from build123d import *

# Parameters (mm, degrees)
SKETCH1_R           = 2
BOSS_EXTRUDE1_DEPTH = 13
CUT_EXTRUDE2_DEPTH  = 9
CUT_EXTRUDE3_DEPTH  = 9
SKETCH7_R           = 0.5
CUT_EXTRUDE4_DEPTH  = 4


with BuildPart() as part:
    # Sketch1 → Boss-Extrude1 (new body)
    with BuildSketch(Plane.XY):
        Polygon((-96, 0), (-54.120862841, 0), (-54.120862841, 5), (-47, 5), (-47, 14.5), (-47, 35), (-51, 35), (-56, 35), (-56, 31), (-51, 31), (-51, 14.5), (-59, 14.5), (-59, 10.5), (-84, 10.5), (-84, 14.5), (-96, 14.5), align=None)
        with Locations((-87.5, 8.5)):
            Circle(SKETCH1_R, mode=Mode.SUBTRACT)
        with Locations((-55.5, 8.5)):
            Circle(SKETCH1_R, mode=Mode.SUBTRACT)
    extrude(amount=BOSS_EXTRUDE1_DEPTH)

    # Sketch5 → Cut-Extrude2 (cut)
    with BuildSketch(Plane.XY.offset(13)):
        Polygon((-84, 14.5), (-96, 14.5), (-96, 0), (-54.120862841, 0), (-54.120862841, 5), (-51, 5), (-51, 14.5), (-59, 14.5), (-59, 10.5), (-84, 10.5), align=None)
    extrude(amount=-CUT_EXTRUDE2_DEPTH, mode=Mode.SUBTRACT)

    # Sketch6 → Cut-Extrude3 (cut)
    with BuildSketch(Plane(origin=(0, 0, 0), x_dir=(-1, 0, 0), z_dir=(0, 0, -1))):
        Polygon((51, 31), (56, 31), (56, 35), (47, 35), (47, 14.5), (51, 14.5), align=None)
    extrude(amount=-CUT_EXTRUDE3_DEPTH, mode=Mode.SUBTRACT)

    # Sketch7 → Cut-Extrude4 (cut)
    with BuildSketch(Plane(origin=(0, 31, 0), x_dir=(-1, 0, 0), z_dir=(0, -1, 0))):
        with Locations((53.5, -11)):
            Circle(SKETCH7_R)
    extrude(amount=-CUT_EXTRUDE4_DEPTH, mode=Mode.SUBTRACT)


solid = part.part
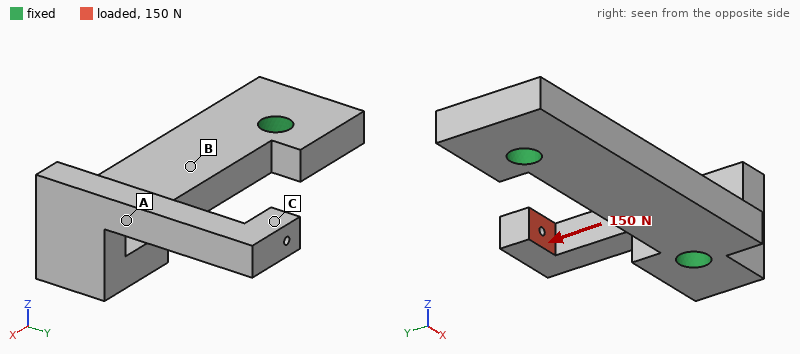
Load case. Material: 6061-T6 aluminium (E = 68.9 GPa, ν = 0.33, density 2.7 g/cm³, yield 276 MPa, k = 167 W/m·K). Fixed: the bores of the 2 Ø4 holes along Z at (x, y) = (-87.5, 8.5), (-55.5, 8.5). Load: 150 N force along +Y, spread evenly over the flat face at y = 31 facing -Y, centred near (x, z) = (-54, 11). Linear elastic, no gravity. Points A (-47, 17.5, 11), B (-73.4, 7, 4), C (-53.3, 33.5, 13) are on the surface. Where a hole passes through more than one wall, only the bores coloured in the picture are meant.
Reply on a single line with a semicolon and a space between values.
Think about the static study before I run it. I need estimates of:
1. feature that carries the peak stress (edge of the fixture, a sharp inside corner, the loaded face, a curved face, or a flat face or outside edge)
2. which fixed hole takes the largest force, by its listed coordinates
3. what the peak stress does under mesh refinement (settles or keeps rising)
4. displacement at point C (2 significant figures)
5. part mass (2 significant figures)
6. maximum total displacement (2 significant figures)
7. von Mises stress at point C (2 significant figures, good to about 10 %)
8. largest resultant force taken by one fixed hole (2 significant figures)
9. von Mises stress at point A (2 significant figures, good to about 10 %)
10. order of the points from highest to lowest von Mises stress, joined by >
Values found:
edge of the fixture; (-55.5, 8.5); keeps rising; 0.16 mm; 8.0 g; 0.19 mm; 16 MPa; 150 N; 53 MPa; A > C > B
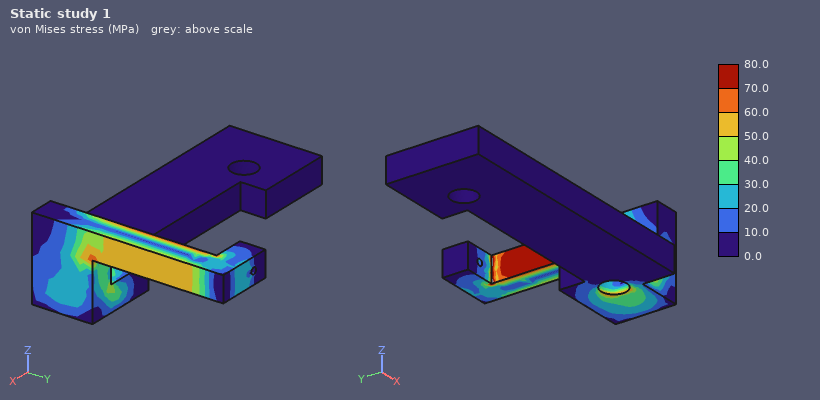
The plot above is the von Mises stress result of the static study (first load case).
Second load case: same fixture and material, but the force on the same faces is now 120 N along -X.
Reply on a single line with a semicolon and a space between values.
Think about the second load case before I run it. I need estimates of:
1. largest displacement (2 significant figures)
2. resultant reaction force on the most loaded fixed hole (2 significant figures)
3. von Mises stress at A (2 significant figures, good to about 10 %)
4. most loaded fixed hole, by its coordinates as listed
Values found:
0.43 mm; 150 N; 150 MPa; (-55.5, 8.5)
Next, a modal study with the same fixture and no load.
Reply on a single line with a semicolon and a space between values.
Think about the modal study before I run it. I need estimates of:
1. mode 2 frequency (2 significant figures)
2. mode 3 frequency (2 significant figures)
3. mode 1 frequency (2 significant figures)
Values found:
4000 Hz; 11 kHz; 3500 Hz
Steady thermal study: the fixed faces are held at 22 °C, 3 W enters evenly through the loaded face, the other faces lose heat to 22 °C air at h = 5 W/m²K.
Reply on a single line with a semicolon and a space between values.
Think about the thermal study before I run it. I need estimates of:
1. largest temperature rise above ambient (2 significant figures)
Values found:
33 K
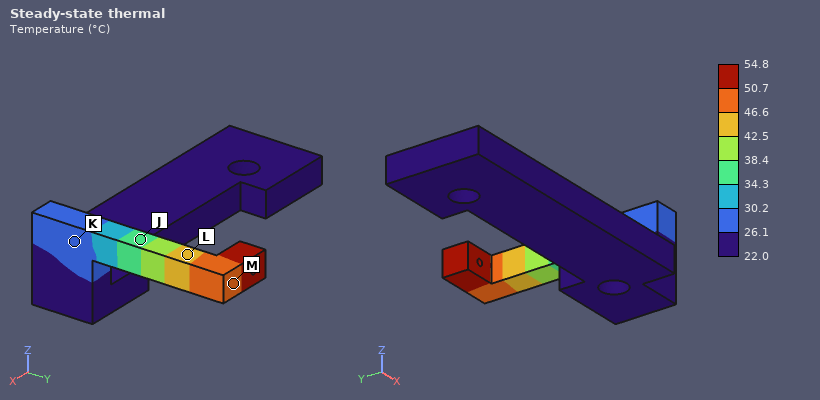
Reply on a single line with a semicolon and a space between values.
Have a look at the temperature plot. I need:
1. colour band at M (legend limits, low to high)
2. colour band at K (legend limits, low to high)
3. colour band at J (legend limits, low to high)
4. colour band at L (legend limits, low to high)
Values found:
46.6 to 50.7 °C; 26.1 to 30.2 °C; 34.3 to 38.4 °C; 42.5 to 46.6 °C
